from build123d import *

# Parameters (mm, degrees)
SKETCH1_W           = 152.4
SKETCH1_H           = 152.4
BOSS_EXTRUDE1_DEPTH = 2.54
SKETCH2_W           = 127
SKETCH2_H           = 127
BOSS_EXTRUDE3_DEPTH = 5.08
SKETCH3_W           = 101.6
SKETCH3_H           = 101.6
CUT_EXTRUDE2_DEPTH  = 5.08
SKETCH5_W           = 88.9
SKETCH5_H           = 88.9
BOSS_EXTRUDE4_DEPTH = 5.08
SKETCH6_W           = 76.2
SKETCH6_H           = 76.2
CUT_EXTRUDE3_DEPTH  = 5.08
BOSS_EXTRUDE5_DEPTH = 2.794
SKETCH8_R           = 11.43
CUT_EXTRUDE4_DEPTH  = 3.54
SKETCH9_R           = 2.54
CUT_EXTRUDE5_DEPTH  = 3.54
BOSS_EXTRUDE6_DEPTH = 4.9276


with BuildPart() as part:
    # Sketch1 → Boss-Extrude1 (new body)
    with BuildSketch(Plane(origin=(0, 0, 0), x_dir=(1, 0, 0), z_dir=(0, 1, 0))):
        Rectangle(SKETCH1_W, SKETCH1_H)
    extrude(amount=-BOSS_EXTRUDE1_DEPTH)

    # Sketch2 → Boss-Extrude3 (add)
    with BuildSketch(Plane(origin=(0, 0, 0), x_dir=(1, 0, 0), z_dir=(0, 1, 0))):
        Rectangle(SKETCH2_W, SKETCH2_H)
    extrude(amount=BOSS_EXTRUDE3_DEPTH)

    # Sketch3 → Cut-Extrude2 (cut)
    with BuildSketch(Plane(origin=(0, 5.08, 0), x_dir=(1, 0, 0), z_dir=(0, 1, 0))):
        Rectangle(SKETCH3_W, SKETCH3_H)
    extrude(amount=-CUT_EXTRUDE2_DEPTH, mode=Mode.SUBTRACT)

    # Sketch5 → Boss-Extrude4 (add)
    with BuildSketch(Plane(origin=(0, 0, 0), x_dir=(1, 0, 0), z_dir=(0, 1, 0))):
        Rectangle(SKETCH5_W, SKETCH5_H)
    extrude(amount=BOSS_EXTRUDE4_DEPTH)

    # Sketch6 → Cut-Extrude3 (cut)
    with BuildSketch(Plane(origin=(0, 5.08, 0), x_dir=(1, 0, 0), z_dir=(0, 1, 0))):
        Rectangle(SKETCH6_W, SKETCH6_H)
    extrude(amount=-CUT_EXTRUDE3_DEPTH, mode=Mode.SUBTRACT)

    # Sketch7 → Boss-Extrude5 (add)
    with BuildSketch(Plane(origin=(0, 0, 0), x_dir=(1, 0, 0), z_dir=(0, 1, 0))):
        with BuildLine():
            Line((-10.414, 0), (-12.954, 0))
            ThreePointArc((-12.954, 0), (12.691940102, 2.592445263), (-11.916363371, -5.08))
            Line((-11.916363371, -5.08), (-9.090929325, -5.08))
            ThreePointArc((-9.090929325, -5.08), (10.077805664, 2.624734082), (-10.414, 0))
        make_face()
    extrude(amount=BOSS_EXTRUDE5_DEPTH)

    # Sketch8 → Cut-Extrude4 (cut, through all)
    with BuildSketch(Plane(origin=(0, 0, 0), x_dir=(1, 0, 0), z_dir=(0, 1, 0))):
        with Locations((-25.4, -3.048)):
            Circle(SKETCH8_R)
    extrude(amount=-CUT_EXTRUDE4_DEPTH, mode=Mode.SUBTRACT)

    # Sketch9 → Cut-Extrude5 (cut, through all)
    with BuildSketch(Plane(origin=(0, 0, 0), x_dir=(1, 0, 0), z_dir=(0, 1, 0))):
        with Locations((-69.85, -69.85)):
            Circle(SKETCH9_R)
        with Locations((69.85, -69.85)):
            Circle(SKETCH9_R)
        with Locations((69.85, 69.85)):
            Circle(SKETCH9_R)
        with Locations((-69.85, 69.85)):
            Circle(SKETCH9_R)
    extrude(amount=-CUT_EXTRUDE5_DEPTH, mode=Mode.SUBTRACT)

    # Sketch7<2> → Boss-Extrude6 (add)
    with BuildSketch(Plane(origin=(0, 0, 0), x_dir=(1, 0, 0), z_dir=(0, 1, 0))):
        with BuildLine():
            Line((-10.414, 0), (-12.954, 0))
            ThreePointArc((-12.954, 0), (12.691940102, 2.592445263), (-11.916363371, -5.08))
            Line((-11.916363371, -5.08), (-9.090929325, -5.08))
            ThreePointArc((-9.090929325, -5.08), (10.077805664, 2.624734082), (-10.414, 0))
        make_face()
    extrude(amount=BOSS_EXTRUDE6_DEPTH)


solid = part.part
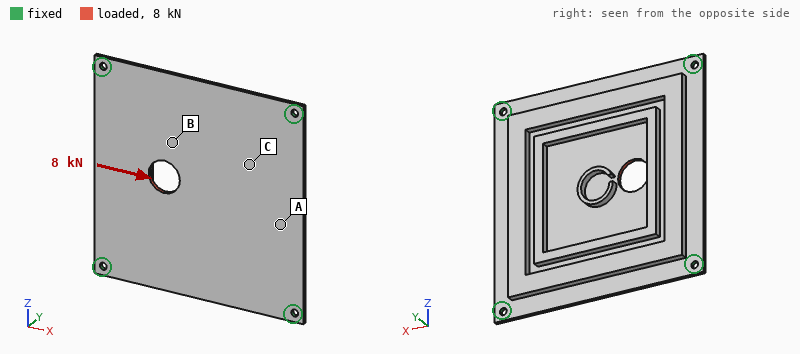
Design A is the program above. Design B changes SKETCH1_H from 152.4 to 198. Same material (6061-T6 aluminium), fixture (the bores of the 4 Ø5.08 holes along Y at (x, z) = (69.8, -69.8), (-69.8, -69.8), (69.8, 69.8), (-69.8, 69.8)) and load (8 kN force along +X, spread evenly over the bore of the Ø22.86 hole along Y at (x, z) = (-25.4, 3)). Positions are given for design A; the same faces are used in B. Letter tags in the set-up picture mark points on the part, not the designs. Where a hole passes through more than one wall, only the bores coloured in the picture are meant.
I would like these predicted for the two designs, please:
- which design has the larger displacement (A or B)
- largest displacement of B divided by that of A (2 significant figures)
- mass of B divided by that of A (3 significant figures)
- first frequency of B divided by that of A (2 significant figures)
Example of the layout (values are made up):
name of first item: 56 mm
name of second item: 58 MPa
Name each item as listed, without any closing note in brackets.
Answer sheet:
which design has the larger displacement: A
largest displacement of B divided by that of A: 0.91
mass of B divided by that of A: 1.18
first frequency of B divided by that of A: 1.0
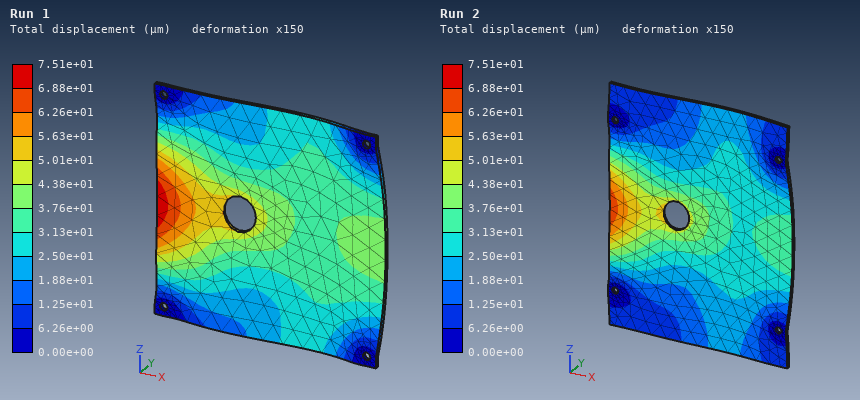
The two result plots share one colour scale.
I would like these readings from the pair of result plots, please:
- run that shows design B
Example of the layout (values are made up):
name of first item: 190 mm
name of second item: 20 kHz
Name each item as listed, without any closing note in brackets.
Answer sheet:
run that shows design B: Run 2
